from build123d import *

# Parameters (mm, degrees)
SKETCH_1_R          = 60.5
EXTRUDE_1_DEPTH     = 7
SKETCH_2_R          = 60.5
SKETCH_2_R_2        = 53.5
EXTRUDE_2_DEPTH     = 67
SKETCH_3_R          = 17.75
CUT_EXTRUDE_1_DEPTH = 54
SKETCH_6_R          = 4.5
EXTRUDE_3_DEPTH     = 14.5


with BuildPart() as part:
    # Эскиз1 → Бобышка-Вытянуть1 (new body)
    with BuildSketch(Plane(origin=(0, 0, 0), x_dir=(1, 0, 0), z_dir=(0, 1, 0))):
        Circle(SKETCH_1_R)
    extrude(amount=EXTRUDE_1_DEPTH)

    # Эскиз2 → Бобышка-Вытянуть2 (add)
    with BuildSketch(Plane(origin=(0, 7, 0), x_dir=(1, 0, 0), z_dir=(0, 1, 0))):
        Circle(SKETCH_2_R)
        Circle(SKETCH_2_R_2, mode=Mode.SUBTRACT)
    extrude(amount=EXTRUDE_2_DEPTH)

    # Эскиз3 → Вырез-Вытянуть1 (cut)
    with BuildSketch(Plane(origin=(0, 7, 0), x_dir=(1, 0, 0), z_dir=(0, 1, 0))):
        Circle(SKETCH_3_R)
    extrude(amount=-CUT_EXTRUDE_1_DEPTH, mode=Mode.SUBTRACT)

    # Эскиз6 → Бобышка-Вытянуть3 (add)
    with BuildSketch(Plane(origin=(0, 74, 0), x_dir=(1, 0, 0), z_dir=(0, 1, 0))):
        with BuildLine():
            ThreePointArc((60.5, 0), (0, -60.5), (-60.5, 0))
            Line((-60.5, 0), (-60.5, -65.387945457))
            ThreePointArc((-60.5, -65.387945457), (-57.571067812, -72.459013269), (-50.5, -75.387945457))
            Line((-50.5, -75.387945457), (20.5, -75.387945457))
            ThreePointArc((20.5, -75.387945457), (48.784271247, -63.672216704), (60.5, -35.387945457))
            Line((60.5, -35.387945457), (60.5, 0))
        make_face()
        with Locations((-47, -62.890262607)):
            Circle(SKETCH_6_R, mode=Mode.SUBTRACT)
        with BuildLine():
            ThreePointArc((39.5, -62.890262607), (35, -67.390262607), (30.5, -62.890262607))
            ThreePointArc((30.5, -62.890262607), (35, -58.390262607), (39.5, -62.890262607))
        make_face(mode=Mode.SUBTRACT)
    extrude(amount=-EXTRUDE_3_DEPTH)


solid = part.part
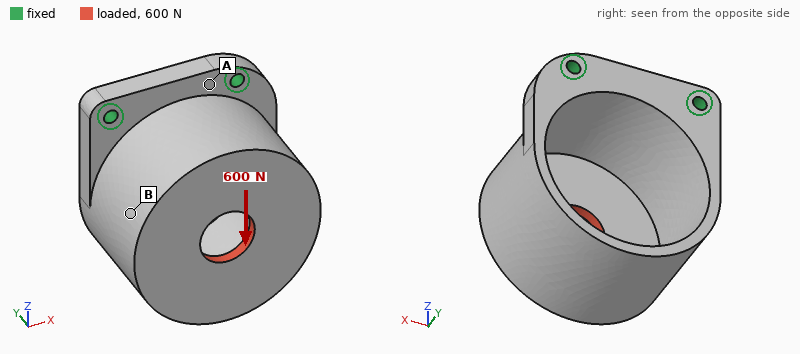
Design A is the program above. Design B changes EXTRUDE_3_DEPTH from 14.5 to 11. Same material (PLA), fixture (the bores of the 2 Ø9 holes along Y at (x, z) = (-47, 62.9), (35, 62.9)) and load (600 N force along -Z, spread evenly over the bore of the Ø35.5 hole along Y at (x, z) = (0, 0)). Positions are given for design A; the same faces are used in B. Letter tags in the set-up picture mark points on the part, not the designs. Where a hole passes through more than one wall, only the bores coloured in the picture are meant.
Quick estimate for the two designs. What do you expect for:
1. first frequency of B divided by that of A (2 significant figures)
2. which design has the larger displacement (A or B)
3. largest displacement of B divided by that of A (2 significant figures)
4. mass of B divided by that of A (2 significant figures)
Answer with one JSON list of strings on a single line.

["0.75", "B", "1.8", "0.96"]
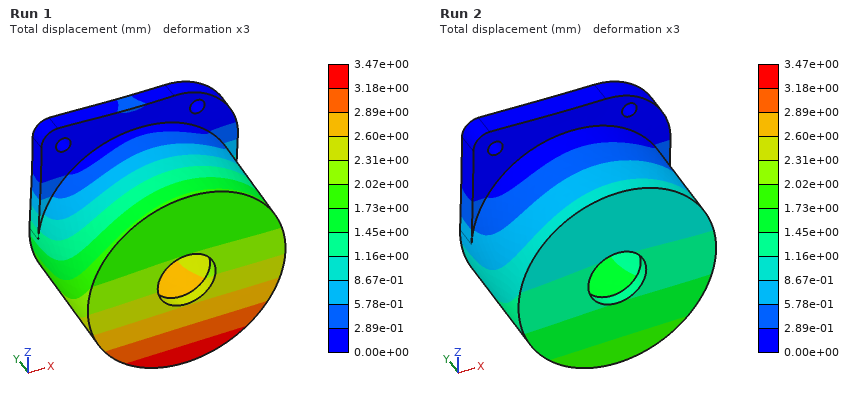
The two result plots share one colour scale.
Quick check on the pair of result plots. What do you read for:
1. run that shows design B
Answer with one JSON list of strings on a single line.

["Run 1"]
